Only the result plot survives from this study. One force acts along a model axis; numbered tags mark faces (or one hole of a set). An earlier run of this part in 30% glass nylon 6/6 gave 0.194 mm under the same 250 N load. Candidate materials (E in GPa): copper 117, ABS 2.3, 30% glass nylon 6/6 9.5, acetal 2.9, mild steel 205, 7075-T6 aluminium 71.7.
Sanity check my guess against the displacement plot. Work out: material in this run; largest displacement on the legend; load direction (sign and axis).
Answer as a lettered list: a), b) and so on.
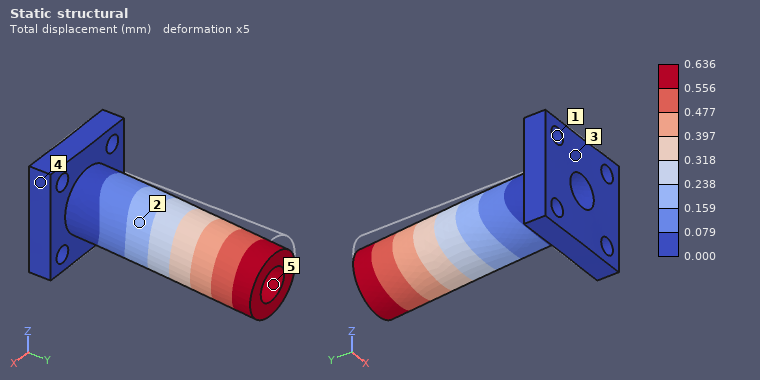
a) acetal
b) 0.636 mm
c) -Z
